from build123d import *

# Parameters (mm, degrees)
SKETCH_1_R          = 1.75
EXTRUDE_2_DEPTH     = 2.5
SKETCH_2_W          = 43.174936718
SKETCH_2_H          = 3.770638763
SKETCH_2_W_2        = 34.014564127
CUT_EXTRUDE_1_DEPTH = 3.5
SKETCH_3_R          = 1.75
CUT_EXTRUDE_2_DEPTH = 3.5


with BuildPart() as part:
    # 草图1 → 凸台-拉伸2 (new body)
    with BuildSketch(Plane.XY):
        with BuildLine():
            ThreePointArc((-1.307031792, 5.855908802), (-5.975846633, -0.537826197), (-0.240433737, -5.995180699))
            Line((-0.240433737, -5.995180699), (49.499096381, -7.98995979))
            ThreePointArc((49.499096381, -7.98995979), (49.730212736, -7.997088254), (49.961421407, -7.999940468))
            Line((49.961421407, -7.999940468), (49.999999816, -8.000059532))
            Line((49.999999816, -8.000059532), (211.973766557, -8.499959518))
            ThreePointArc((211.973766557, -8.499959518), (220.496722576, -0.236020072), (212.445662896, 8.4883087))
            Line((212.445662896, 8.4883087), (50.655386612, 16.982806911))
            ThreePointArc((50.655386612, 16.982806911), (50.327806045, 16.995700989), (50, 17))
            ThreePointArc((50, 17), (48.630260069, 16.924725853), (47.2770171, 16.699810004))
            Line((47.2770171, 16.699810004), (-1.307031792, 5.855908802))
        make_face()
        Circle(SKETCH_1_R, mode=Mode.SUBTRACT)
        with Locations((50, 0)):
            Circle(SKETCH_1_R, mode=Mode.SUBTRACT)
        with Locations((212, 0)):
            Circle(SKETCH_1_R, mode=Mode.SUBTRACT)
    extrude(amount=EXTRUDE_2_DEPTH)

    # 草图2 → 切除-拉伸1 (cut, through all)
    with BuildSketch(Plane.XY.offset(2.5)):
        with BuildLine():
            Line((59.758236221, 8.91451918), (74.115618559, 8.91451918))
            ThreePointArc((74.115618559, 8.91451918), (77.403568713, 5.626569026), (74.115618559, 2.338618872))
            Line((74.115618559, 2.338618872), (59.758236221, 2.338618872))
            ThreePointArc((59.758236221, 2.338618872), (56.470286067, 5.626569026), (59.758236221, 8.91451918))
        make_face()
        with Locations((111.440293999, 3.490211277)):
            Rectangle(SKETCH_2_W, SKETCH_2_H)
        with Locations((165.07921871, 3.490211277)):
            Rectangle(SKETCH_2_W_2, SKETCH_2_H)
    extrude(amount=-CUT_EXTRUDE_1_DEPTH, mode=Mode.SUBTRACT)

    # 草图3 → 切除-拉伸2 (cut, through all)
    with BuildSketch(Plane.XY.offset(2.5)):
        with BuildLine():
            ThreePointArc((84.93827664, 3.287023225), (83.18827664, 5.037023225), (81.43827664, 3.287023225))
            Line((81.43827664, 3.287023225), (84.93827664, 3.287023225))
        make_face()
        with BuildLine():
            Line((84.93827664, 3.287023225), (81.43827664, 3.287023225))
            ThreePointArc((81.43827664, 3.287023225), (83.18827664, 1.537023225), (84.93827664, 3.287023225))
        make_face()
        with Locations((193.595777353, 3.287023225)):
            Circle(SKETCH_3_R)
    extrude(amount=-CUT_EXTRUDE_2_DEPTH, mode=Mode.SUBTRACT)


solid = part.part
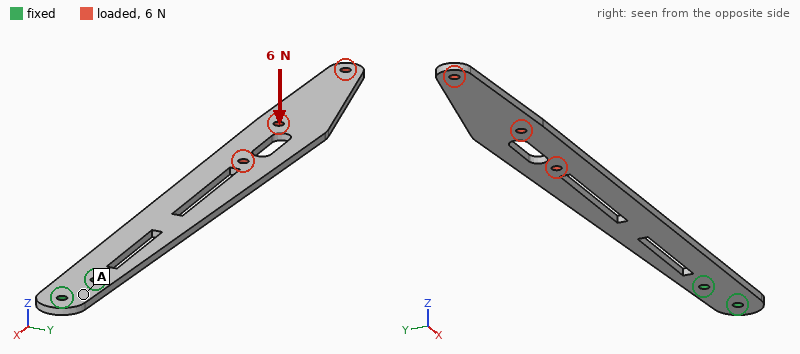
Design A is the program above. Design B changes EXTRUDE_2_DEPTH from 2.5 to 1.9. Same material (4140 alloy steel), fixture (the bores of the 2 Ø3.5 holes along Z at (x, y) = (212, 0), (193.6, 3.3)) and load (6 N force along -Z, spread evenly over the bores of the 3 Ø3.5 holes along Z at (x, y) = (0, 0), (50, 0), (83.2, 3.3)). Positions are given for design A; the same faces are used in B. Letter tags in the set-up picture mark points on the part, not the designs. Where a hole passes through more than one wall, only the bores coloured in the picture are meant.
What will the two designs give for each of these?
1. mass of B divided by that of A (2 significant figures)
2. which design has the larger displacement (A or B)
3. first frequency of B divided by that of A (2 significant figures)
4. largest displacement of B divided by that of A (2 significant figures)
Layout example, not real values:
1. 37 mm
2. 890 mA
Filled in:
1. 0.76
2. B
3. 0.76
4. 2.3
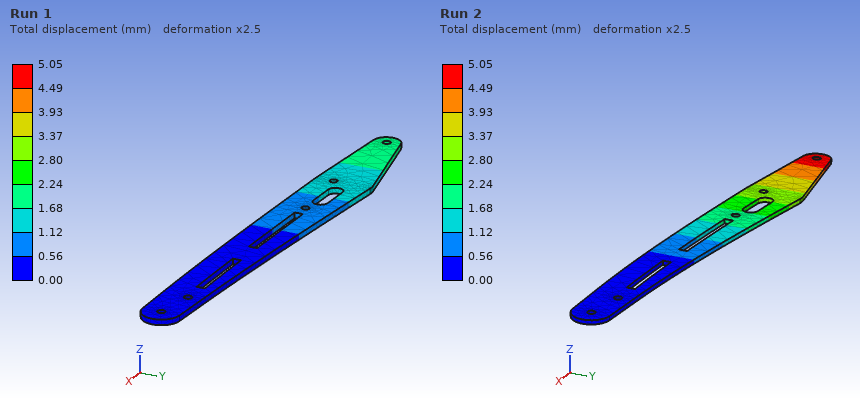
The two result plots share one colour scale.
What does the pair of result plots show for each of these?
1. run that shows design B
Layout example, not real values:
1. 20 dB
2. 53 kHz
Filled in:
1. Run 2
